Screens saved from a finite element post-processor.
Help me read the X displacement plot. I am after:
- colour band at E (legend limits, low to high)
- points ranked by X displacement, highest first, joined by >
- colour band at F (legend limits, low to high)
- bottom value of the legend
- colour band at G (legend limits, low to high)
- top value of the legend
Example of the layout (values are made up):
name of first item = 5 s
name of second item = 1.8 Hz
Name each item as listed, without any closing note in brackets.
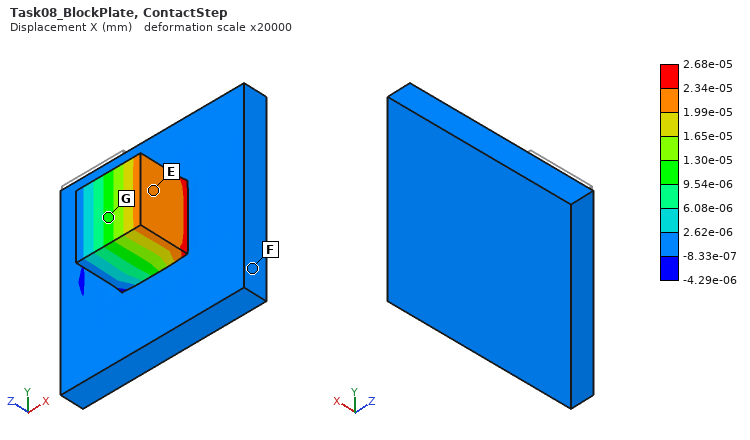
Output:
colour band at E = 1.99e-05 to 2.34e-05 mm
points ranked by X displacement, highest first, joined by > = E > G > F
colour band at F = -8.33e-07 to 2.62e-06 mm
bottom value of the legend = -4.29e-06 mm
colour band at G = 9.54e-06 to 1.30e-05 mm
top value of the legend = 2.68e-05 mm
